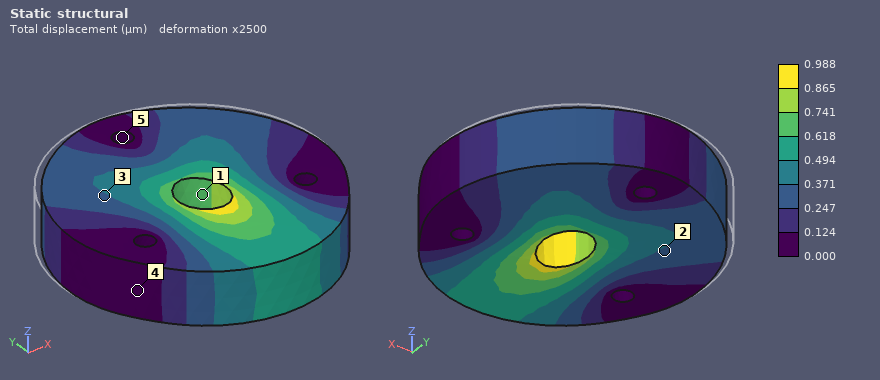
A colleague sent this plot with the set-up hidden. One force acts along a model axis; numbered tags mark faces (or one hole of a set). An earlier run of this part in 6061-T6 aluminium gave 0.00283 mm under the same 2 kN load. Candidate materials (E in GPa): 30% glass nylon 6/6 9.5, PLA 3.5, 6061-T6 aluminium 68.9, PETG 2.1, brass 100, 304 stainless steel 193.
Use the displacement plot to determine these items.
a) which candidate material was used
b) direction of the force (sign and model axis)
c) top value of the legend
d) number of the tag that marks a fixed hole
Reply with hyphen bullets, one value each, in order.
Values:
- 304 stainless steel
- -Y
- 0.988 µm
- 5
